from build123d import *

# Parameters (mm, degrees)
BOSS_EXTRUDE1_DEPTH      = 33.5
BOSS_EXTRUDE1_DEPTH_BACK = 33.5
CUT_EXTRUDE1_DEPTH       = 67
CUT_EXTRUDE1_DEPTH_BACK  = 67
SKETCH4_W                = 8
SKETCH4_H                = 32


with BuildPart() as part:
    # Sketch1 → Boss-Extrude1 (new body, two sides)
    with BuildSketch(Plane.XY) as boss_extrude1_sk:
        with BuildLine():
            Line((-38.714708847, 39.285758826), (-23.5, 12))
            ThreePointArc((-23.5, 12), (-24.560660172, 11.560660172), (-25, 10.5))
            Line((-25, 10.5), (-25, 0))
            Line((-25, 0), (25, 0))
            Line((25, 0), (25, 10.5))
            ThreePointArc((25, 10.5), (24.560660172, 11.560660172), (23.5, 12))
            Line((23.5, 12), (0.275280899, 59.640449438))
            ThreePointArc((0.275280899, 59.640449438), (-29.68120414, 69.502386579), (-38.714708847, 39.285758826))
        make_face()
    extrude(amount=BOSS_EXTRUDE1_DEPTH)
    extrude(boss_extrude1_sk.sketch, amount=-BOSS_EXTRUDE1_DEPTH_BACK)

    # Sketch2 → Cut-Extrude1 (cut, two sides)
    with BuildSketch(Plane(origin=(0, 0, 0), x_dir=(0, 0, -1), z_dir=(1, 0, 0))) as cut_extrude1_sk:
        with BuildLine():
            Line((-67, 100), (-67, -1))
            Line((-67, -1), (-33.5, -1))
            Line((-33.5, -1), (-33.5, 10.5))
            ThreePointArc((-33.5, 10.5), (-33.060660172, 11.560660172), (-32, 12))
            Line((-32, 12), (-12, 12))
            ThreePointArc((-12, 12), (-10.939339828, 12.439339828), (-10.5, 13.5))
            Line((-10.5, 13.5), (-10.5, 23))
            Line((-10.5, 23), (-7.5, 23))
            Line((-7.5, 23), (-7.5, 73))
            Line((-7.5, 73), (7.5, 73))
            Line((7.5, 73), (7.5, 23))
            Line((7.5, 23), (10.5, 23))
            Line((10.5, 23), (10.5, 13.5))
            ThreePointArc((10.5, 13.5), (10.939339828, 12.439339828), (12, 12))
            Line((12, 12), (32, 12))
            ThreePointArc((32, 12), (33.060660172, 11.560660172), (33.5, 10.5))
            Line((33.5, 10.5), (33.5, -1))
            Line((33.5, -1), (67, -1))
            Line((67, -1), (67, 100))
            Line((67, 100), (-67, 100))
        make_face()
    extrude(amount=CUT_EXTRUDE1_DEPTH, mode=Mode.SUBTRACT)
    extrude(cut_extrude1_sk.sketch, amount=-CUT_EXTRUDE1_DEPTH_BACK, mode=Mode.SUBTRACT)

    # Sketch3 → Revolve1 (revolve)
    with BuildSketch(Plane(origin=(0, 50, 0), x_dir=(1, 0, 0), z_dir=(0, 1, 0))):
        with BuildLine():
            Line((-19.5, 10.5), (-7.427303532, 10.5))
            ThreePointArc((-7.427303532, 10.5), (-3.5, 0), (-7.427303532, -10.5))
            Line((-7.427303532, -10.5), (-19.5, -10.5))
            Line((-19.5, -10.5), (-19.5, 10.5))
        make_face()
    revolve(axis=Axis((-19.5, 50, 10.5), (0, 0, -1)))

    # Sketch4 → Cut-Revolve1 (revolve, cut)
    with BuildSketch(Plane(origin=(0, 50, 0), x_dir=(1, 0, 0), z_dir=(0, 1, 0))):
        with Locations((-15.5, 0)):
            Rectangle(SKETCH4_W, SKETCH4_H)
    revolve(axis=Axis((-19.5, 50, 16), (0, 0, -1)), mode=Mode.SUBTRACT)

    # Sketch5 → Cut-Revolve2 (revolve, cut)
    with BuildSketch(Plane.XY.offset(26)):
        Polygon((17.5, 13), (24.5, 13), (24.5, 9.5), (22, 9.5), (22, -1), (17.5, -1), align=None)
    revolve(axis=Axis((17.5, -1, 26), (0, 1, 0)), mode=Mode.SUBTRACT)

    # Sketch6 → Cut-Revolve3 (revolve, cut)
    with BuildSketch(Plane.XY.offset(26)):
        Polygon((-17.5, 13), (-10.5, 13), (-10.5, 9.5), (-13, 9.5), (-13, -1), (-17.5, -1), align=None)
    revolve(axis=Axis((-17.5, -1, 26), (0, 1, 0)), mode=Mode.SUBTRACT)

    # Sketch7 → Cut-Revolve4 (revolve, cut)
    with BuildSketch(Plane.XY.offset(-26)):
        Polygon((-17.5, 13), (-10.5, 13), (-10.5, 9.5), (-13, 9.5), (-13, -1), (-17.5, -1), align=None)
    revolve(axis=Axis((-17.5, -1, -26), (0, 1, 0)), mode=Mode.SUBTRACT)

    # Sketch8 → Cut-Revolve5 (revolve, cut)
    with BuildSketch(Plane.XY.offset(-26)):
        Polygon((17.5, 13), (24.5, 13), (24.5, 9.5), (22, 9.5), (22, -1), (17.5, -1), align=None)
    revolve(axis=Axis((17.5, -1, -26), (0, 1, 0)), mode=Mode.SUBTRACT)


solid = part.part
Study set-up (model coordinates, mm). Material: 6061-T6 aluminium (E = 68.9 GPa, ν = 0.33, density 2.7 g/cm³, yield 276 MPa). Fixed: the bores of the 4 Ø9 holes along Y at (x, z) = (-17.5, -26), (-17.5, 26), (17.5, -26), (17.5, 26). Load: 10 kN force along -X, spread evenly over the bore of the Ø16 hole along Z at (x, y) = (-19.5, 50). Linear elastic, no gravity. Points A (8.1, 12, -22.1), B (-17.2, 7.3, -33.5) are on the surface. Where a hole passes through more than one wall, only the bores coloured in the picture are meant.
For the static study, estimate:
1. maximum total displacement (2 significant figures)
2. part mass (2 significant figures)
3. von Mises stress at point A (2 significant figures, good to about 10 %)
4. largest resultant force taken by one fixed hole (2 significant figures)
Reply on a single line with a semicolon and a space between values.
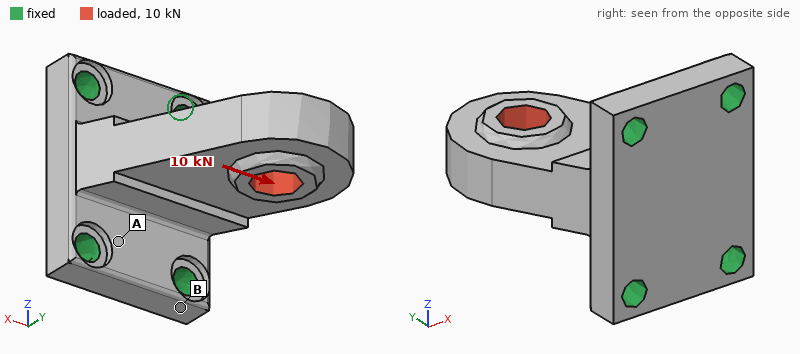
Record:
0.22 mm; 210 g; 45 MPa; 7.5 kN
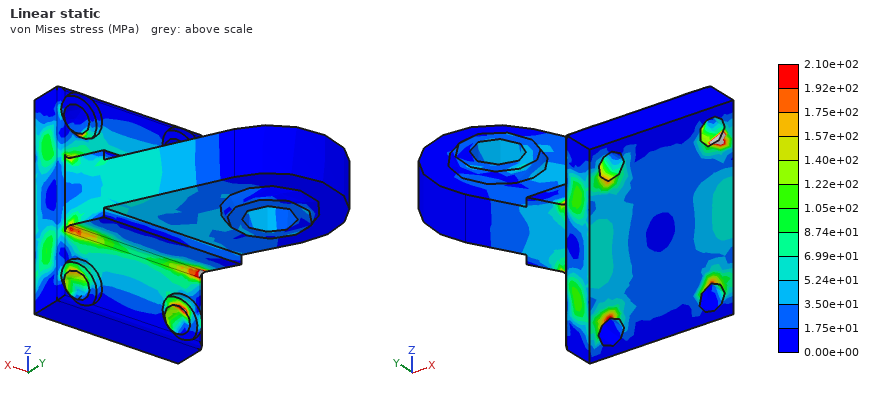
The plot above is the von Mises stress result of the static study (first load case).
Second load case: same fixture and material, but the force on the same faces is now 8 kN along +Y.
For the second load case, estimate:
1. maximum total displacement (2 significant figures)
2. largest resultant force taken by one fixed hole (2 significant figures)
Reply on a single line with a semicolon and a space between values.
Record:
79 µm; 4.5 kN
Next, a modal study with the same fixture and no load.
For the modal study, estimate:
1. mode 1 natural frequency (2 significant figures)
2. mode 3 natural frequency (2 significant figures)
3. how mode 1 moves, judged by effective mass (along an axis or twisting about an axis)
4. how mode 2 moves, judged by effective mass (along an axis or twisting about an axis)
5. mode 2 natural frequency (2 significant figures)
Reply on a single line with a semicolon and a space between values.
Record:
3600 Hz; 9300 Hz; along Z; along X; 4500 Hz
